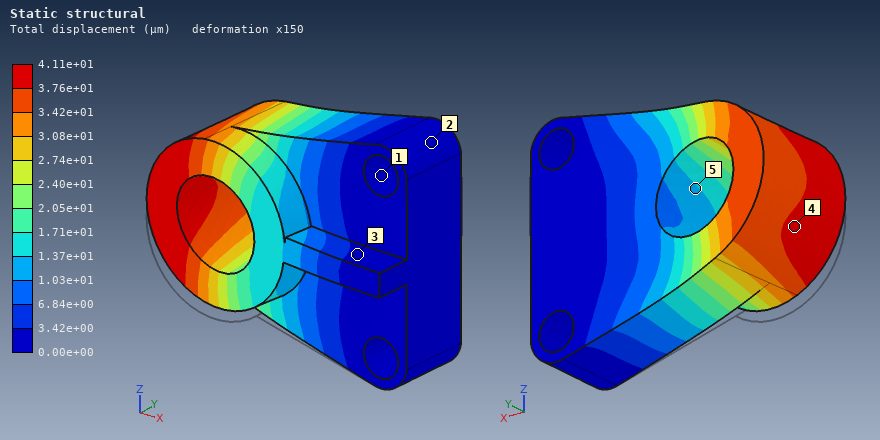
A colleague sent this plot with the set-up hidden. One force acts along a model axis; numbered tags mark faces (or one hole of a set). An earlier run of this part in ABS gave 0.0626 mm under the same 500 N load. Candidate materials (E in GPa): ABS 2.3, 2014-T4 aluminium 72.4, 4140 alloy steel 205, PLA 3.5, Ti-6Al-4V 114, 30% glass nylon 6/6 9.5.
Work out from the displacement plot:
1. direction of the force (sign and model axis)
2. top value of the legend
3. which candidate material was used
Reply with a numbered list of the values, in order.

1. +Z
2. 4.11e+01 µm
3. PLA
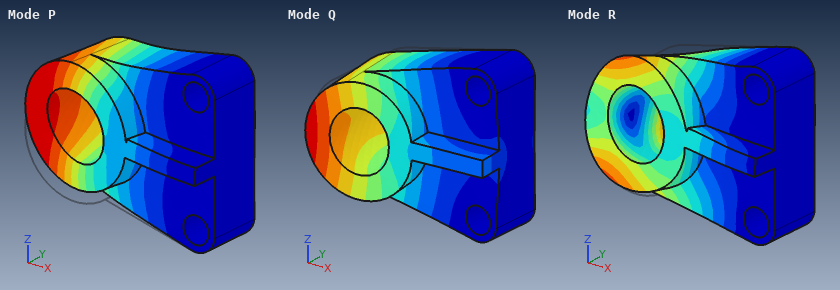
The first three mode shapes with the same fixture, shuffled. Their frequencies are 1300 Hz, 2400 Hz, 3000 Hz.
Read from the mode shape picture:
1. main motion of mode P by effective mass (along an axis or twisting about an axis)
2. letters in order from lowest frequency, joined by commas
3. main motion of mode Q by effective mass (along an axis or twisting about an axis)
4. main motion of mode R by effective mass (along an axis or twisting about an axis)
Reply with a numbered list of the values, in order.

1. along Z
2. Q, P, R
3. along Y
4. twisting about X
